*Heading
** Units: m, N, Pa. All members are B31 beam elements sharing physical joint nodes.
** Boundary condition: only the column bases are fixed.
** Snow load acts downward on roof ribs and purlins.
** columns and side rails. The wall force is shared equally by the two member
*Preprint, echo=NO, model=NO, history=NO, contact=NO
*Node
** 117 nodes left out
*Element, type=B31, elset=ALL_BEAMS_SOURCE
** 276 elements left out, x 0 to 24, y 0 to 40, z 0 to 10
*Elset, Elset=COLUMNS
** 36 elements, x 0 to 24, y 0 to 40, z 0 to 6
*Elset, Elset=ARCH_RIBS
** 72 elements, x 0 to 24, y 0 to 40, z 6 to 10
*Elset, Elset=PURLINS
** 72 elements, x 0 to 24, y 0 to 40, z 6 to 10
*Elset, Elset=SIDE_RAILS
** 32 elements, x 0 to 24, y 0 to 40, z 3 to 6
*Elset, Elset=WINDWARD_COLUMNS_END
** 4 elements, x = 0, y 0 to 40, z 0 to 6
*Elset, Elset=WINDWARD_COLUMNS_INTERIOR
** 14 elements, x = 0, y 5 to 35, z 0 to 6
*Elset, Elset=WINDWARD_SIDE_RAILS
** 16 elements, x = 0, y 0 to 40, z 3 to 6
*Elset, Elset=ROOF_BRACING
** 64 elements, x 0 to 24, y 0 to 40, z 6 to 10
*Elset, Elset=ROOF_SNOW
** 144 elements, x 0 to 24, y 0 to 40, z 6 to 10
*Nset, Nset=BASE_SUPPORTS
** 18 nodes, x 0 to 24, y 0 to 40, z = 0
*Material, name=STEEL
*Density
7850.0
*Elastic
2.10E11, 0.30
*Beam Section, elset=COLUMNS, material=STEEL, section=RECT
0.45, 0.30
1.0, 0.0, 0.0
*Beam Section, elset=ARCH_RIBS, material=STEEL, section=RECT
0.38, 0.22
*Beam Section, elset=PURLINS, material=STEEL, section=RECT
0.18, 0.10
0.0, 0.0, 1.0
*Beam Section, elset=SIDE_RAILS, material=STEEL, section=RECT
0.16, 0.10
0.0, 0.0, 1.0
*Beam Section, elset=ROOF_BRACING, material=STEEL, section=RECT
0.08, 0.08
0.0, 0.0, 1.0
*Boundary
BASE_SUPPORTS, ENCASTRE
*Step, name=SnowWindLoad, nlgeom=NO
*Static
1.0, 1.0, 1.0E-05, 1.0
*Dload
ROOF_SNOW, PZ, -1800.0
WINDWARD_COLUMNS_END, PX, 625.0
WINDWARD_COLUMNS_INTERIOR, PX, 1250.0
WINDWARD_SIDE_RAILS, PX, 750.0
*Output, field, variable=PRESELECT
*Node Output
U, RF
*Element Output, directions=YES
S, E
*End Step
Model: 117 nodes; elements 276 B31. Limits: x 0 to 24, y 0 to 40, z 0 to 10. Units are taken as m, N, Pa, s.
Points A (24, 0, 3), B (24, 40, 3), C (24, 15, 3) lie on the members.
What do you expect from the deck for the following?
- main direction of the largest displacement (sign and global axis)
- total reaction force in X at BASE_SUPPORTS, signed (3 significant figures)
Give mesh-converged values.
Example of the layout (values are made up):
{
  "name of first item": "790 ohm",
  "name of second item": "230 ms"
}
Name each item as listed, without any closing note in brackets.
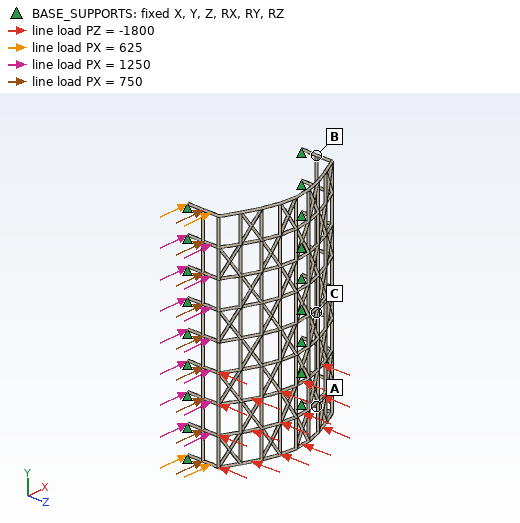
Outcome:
{
  "main direction of the largest displacement": "-Z",
  "total reaction force in X at BASE_SUPPORTS, signed": "-1.20e+05 N"
}
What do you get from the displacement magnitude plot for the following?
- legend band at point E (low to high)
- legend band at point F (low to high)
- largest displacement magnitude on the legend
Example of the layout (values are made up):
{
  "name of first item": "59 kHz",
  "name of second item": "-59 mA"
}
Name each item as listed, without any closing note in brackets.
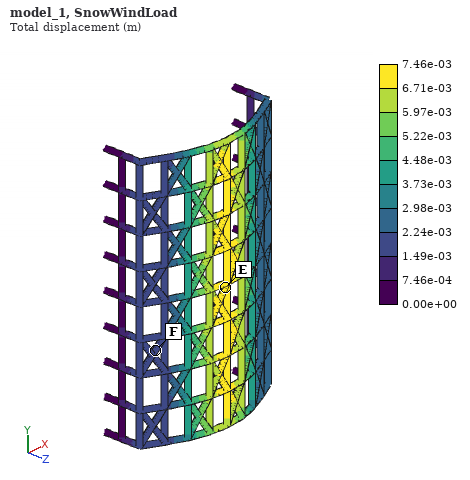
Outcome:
{
  "legend band at point E": "6.71e-03 to 7.46e-03 m",
  "legend band at point F": "1.49e-03 to 2.24e-03 m",
  "largest displacement magnitude on the legend": "7.46e-03 m"
}
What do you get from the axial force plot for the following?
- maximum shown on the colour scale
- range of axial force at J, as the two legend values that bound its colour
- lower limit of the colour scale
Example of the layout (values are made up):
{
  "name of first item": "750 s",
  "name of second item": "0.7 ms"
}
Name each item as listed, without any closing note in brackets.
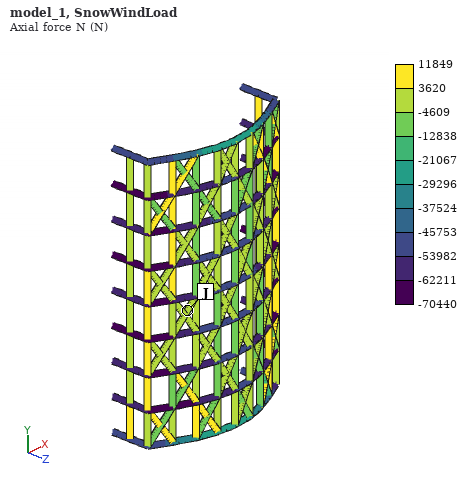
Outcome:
{
  "maximum shown on the colour scale": "11849 N",
  "range of axial force at J, as the two legend values that bound its colour": "-4609 to 3620 N",
  "lower limit of the colour scale": "-70440 N"
}
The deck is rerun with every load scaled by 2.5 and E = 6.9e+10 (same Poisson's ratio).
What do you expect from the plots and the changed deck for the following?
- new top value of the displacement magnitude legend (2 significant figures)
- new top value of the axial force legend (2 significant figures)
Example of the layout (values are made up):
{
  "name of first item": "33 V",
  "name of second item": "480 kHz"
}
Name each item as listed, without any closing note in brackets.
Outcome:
{
  "new top value of the displacement magnitude legend": "0.057 m",
  "new top value of the axial force legend": "30000 N"
}
